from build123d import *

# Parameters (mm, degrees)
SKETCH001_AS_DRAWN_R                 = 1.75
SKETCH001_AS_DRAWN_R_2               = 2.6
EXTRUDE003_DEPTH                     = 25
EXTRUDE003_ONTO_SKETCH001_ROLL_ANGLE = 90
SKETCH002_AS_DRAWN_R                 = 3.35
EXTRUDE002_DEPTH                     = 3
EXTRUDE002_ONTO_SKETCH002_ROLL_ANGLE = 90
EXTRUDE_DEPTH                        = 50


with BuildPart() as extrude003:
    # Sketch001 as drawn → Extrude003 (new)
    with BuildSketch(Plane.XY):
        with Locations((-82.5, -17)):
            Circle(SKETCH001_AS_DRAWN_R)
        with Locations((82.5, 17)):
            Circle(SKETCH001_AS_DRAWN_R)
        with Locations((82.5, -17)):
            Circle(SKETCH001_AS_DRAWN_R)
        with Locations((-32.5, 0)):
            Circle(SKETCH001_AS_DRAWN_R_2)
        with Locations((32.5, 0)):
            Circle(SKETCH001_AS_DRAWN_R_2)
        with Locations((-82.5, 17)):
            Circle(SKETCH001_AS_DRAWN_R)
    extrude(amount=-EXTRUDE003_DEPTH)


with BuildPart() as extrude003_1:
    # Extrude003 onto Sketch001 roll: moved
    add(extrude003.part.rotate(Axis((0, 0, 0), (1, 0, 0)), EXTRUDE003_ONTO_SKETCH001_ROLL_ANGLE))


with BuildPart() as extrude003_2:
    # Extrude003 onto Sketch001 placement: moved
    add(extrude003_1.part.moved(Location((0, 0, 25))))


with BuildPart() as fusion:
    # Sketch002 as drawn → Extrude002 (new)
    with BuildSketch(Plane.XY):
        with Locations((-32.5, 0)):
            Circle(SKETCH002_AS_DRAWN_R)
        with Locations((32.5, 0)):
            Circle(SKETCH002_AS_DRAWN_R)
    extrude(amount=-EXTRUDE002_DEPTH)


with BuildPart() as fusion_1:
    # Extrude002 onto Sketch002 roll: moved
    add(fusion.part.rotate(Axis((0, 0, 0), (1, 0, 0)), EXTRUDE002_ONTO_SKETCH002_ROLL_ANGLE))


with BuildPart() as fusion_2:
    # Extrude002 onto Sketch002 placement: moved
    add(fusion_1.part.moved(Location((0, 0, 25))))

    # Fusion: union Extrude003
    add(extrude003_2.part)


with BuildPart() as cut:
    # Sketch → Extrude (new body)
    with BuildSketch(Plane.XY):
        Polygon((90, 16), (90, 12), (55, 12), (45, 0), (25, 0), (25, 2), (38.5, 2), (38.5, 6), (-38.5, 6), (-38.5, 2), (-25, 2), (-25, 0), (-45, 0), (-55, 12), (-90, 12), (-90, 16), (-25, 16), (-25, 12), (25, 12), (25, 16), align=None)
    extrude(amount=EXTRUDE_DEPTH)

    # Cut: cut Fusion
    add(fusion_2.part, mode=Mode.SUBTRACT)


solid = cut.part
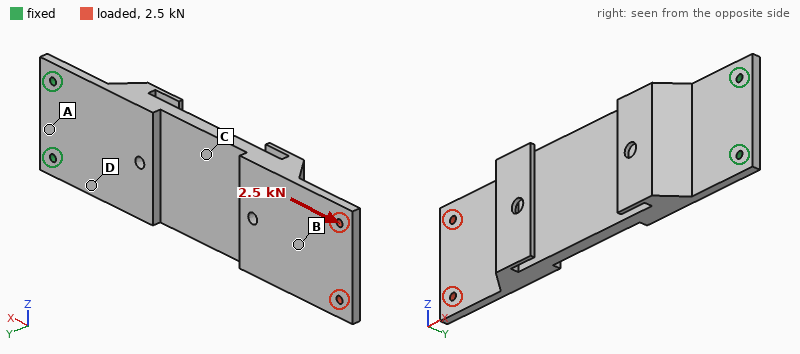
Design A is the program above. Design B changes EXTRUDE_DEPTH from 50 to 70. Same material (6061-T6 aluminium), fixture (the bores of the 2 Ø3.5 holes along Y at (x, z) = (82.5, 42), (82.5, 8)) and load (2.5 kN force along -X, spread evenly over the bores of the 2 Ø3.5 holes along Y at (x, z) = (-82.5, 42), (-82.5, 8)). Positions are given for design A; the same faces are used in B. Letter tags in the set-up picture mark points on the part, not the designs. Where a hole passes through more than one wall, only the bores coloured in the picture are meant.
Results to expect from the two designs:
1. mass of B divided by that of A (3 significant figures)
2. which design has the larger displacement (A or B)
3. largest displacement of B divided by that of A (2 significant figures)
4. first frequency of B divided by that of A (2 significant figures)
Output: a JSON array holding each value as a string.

["1.40", "A", "0.71", "0.95"]
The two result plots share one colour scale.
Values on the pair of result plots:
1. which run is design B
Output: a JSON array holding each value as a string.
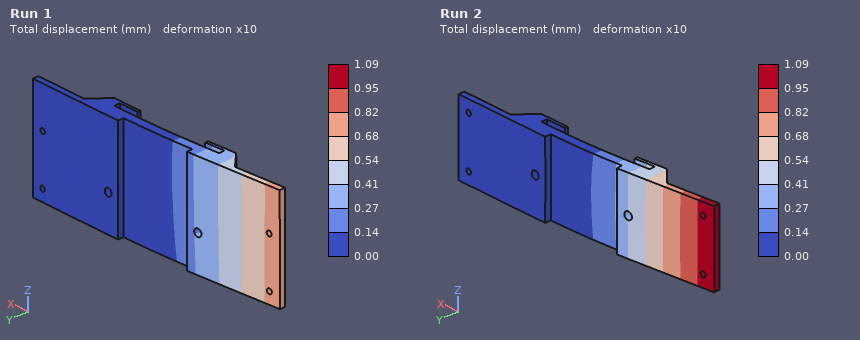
["Run 1"]
